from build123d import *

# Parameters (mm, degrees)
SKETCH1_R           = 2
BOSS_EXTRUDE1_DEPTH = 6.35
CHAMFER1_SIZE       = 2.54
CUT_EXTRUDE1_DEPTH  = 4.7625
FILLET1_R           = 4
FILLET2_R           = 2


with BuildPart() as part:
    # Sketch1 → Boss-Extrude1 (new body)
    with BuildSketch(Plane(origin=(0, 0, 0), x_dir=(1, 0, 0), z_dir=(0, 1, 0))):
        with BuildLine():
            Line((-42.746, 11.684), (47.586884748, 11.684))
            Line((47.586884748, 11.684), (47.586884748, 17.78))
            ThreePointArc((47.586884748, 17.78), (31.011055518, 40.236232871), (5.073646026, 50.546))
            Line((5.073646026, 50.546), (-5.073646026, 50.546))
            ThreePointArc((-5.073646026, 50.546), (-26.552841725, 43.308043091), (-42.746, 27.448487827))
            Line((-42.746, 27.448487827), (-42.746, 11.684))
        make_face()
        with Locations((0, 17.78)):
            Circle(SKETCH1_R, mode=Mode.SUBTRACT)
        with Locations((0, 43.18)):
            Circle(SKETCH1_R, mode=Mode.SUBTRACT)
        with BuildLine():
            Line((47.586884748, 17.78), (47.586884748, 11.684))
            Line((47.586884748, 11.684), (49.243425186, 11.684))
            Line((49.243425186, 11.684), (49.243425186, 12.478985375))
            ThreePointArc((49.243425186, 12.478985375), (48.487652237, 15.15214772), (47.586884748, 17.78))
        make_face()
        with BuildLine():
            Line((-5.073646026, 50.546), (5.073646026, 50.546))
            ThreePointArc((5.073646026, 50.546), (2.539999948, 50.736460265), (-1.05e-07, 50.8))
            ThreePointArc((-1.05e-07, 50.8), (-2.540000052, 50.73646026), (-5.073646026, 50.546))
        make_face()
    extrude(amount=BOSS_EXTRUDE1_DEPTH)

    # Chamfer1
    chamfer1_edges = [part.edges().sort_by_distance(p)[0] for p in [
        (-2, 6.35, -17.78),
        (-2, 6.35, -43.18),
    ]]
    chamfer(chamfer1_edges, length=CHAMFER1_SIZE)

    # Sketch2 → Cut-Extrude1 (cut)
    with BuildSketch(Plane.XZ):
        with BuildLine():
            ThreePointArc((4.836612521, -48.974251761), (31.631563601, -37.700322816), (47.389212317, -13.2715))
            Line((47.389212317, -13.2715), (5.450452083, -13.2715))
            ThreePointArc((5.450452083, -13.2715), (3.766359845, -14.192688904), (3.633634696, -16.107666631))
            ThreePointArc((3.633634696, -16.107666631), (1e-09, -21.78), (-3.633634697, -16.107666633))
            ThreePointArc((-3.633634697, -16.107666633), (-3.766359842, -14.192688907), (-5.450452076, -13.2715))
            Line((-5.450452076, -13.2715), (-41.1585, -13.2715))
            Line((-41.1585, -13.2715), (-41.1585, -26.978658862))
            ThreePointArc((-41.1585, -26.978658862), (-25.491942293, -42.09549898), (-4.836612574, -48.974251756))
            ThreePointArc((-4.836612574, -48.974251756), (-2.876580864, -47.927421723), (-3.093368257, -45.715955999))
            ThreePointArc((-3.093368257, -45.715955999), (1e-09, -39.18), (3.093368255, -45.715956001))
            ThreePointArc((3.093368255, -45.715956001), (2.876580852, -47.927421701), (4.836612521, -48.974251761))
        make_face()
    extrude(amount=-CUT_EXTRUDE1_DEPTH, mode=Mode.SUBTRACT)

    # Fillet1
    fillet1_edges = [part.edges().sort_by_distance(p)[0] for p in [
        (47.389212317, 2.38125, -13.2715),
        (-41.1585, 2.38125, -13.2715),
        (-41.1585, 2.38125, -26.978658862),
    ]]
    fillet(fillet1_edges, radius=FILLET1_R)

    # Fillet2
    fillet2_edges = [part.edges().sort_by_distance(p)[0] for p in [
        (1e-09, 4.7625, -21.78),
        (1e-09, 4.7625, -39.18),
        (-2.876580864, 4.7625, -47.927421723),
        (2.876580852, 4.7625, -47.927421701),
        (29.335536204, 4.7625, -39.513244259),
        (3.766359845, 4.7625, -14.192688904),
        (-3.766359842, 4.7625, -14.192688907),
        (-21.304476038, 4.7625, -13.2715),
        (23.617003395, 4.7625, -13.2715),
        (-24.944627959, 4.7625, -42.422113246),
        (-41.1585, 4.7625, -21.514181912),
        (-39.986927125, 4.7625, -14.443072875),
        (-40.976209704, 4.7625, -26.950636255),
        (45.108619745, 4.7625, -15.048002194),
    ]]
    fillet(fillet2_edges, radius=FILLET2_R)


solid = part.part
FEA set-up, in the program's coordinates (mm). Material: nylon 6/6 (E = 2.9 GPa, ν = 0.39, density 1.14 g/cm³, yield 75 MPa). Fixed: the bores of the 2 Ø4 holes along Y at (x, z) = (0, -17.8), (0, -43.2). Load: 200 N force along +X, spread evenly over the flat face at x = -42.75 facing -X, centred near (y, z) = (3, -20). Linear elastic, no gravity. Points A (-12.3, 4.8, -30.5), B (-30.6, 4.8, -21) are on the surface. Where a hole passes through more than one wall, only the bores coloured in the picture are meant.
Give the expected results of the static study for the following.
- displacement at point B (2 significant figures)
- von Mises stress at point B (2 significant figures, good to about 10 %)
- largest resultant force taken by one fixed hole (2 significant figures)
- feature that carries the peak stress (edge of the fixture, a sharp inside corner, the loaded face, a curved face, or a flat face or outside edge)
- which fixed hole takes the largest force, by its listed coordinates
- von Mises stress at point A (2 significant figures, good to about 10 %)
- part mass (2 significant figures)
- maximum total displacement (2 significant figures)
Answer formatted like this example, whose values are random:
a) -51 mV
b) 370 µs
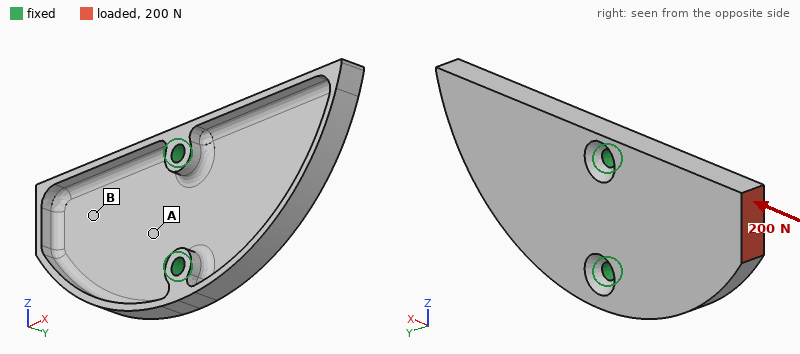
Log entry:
a) 0.34 mm
b) 7.6 MPa
c) 170 N
d) a curved face
e) (0, -17.8)
f) 3.5 MPa
g) 7.7 g
h) 1.0 mm
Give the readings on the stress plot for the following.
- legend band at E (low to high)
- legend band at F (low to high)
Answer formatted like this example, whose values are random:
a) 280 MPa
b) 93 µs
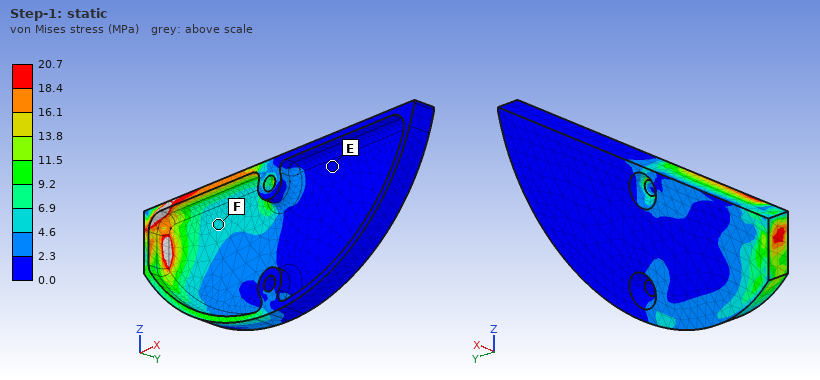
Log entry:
a) 0.0 to 2.3 MPa
b) 4.6 to 6.9 MPa
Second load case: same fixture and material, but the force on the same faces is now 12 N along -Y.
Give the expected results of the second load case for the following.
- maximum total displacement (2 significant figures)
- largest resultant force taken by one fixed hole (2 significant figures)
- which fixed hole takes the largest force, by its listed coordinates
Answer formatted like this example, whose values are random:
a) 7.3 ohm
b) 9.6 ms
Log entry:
a) 1.00 mm
b) 8.7 N
c) (0, -17.8)
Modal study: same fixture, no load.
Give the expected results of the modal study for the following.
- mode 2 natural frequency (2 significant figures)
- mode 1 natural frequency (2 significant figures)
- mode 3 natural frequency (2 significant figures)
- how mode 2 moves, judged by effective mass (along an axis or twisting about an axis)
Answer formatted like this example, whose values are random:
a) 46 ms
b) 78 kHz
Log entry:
a) 650 Hz
b) 510 Hz
c) 1300 Hz
d) along Y
